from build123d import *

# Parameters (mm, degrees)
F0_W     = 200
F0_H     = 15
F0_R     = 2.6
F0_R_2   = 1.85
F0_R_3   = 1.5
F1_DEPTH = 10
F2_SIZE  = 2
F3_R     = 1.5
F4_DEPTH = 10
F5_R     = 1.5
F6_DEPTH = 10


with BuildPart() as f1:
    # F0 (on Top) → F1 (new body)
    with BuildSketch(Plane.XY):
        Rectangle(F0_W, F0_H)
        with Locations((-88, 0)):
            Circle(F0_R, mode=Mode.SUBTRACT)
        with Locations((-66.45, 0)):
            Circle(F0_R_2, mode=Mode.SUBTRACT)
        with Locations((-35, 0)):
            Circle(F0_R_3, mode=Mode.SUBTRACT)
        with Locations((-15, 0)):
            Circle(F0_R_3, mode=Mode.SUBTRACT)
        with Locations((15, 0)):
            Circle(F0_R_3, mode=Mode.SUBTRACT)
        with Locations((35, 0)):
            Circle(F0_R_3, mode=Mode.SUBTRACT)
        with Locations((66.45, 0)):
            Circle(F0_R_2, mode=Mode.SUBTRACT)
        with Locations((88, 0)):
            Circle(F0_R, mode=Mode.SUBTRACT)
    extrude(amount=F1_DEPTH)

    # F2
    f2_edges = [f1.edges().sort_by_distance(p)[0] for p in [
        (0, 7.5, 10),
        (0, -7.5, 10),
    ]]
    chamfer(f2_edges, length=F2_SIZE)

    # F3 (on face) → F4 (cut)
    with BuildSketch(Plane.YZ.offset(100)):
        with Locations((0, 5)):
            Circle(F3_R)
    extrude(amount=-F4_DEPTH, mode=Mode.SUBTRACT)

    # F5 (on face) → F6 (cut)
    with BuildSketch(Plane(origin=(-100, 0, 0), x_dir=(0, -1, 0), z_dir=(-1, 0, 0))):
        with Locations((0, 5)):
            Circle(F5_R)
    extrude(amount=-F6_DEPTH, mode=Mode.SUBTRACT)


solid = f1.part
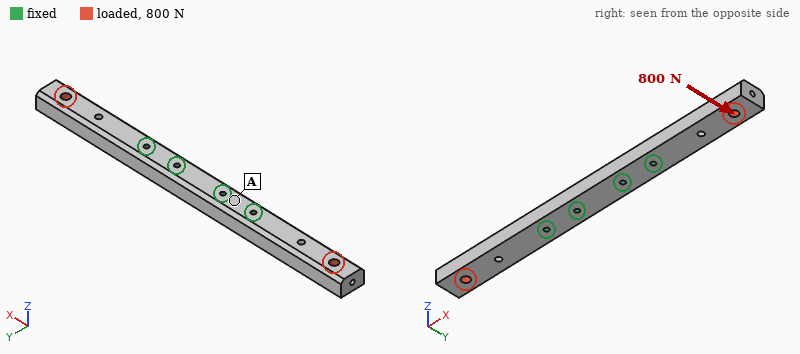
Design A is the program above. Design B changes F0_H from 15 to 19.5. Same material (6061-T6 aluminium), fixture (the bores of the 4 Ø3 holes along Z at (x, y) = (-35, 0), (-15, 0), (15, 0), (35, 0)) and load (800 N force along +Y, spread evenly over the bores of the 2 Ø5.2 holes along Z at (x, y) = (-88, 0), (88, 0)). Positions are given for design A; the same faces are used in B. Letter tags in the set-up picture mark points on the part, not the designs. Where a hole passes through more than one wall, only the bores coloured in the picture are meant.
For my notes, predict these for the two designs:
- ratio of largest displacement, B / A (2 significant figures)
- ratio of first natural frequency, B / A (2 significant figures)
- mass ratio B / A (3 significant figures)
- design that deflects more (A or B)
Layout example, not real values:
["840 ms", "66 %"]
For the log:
["0.51", "0.98", "1.32", "A"]
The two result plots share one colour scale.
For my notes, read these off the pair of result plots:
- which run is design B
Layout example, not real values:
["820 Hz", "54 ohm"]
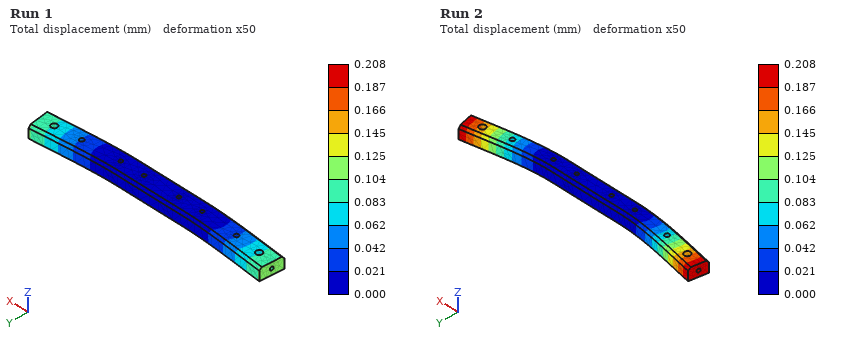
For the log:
["Run 1"]
